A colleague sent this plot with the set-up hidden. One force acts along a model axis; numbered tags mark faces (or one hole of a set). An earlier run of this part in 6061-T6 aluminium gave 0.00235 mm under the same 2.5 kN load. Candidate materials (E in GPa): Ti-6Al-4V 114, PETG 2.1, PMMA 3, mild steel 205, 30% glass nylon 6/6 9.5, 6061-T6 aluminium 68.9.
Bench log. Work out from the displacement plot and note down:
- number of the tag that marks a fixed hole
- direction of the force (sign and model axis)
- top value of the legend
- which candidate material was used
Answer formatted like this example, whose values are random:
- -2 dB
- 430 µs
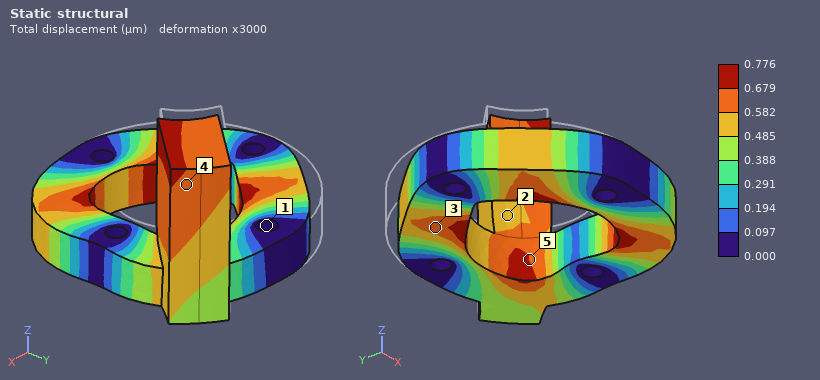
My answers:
- 1
- +X
- 0.776 µm
- mild steel
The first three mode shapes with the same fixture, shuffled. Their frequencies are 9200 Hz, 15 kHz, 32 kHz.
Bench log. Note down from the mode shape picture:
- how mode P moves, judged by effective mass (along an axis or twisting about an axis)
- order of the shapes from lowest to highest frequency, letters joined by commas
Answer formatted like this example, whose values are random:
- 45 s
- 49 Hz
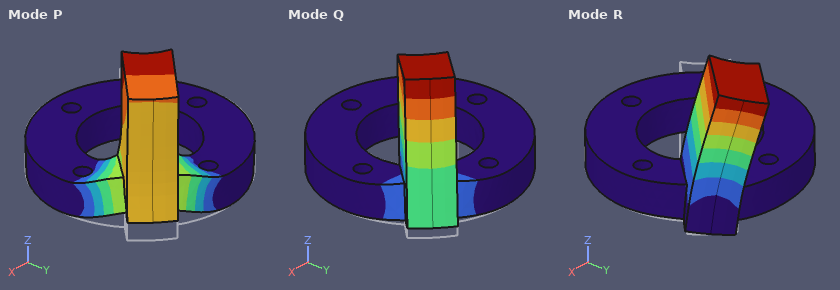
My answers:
- along Z
- Q, R, P
